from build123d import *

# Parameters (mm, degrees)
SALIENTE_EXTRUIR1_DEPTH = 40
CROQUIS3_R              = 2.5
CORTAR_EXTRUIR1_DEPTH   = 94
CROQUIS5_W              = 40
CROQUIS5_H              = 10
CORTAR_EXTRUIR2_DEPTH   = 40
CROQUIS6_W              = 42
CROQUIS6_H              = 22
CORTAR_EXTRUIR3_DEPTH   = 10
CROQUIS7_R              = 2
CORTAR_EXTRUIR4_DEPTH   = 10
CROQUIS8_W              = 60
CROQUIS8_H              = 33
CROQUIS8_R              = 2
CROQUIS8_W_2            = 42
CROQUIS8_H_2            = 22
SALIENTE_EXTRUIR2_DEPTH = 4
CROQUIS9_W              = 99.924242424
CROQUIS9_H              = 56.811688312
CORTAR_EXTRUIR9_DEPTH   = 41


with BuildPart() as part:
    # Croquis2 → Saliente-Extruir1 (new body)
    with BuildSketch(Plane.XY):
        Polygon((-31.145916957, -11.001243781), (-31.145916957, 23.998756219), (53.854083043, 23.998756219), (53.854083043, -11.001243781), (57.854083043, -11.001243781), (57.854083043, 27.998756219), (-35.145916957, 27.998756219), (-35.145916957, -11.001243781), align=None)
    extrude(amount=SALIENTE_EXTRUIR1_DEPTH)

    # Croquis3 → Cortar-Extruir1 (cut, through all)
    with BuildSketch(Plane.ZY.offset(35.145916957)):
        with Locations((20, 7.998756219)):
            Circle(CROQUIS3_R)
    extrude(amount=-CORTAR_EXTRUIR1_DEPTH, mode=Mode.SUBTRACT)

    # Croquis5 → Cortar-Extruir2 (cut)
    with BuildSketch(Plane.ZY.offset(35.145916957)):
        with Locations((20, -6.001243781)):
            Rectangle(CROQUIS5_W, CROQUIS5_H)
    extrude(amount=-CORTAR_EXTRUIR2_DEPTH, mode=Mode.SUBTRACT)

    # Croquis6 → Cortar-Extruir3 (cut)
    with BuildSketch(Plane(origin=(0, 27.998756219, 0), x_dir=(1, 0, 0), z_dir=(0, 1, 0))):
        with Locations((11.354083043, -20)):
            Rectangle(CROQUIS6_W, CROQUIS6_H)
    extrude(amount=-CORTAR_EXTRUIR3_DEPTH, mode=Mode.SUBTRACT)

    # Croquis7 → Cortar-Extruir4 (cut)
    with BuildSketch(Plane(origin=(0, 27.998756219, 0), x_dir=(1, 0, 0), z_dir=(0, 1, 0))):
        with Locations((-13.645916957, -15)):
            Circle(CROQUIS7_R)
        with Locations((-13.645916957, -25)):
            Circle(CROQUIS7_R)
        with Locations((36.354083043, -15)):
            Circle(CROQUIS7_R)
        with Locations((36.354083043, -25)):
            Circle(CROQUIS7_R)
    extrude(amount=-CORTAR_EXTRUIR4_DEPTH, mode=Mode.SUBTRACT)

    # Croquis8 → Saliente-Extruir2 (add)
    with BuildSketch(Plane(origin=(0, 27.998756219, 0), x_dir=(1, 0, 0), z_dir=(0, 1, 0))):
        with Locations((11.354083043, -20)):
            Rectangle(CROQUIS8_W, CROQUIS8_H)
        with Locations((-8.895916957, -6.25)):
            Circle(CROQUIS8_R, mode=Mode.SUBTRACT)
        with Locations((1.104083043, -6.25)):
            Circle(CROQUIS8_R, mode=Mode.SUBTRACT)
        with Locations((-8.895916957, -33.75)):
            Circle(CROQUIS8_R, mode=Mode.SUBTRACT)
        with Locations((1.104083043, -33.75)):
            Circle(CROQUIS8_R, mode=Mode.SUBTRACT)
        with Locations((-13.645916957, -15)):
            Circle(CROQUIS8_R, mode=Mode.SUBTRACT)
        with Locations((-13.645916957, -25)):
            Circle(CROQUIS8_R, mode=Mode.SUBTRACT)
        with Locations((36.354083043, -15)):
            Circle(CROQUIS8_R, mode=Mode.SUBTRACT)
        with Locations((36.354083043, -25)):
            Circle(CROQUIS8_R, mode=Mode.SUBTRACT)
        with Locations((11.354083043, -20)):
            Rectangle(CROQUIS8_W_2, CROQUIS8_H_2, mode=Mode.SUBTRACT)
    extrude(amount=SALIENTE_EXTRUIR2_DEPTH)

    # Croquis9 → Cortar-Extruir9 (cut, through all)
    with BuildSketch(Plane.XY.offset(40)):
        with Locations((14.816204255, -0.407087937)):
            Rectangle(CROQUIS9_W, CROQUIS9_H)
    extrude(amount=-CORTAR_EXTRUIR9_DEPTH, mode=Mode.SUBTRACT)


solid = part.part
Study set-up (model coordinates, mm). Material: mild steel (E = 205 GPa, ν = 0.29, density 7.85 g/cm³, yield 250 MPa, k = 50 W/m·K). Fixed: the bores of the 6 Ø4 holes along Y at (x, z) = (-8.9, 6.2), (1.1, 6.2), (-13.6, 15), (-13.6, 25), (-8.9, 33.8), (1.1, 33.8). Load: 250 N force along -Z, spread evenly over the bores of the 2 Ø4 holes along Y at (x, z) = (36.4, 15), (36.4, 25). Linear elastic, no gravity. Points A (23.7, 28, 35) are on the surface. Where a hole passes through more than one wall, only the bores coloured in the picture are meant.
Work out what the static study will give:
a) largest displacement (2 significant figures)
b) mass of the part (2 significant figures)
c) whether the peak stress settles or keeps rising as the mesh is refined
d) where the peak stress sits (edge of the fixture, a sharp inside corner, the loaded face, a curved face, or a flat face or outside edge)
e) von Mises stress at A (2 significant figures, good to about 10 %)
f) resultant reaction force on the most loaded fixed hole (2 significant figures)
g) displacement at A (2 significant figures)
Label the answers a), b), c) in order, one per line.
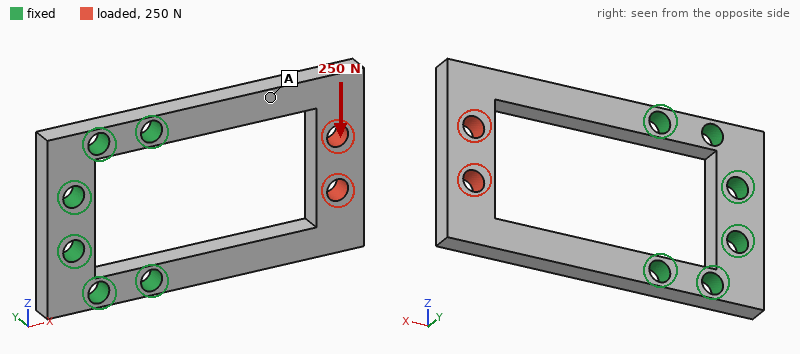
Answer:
a) 42 µm
b) 30 g
c) keeps rising
d) edge of the fixture
e) 14 MPa
f) 200 N
g) 28 µm
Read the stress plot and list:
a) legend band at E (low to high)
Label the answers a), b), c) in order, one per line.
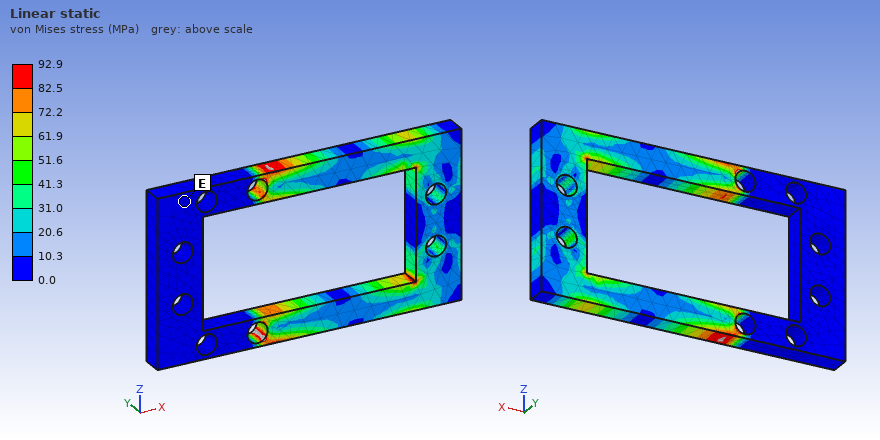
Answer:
a) 0.0 to 10.3 MPa
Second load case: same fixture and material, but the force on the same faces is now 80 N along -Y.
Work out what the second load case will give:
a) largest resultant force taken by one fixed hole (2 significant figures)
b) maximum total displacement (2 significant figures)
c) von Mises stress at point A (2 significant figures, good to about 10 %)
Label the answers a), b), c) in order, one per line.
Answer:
a) 41 N
b) 0.11 mm
c) 34 MPa
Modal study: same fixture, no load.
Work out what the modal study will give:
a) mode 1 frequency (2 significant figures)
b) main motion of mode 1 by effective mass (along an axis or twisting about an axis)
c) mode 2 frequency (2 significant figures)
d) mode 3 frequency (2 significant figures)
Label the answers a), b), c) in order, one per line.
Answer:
a) 1500 Hz
b) along Y
c) 3700 Hz
d) 3800 Hz
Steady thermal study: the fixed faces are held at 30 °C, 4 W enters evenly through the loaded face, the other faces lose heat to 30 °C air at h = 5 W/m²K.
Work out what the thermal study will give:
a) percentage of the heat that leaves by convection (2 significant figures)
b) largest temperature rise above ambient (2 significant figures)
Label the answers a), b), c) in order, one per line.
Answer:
a) 9.5 %
b) 64 K
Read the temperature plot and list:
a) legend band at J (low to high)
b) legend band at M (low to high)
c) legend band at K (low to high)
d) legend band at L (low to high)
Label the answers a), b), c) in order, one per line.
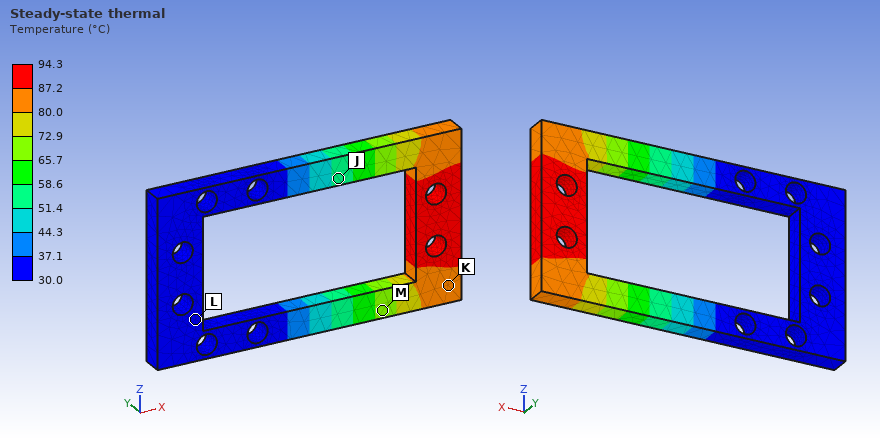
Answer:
a) 51.4 to 58.6 °C
b) 65.7 to 72.9 °C
c) 80.0 to 87.2 °C
d) 30.0 to 37.1 °C
